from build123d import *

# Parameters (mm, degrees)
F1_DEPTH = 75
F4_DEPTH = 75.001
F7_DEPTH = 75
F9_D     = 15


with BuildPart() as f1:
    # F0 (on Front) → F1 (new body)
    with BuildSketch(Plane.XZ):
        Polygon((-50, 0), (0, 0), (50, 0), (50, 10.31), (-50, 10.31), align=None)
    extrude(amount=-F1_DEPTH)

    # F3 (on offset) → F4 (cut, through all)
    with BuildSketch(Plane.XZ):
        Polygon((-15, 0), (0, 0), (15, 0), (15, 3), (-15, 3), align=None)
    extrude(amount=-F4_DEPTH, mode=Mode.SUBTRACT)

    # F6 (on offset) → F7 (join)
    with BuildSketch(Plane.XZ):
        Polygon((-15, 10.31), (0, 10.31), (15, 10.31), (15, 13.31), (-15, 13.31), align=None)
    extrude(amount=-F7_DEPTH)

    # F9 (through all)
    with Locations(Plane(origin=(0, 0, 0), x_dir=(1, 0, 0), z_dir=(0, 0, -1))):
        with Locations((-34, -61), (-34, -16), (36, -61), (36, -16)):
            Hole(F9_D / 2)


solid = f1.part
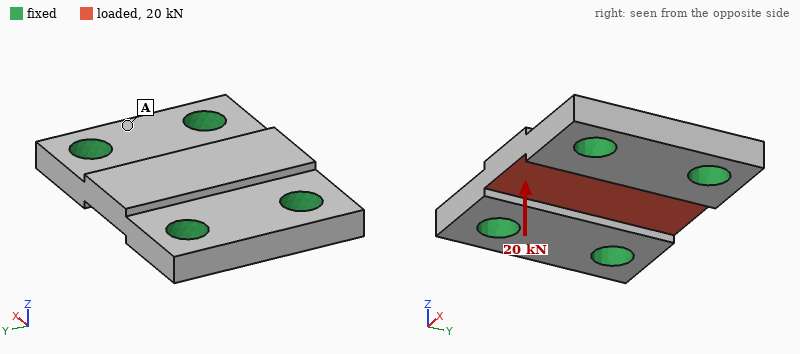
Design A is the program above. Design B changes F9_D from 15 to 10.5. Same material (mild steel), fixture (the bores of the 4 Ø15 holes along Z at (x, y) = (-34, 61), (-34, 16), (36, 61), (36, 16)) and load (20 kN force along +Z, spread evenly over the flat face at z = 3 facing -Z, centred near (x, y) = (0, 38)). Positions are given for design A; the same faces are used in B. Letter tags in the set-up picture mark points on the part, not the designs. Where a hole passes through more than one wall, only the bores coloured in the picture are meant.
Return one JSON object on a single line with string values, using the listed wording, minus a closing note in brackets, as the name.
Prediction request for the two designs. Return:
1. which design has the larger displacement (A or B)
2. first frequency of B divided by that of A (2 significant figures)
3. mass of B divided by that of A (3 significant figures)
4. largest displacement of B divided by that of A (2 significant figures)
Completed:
{"which design has the larger displacement": "B", "first frequency of B divided by that of A": "0.85", "mass of B divided by that of A": "1.05", "largest displacement of B divided by that of A": "1.3"}
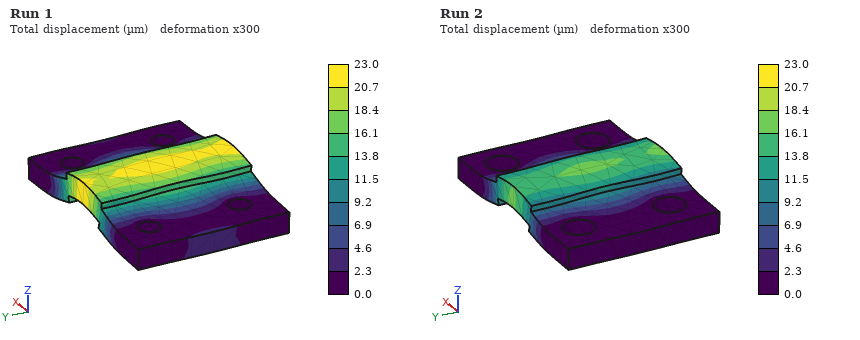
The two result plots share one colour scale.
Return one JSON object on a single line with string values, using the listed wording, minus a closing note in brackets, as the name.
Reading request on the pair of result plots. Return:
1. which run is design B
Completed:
{"which run is design B": "Run 1"}
